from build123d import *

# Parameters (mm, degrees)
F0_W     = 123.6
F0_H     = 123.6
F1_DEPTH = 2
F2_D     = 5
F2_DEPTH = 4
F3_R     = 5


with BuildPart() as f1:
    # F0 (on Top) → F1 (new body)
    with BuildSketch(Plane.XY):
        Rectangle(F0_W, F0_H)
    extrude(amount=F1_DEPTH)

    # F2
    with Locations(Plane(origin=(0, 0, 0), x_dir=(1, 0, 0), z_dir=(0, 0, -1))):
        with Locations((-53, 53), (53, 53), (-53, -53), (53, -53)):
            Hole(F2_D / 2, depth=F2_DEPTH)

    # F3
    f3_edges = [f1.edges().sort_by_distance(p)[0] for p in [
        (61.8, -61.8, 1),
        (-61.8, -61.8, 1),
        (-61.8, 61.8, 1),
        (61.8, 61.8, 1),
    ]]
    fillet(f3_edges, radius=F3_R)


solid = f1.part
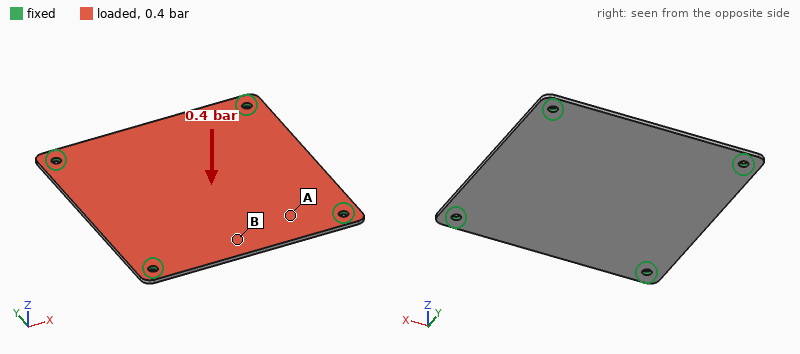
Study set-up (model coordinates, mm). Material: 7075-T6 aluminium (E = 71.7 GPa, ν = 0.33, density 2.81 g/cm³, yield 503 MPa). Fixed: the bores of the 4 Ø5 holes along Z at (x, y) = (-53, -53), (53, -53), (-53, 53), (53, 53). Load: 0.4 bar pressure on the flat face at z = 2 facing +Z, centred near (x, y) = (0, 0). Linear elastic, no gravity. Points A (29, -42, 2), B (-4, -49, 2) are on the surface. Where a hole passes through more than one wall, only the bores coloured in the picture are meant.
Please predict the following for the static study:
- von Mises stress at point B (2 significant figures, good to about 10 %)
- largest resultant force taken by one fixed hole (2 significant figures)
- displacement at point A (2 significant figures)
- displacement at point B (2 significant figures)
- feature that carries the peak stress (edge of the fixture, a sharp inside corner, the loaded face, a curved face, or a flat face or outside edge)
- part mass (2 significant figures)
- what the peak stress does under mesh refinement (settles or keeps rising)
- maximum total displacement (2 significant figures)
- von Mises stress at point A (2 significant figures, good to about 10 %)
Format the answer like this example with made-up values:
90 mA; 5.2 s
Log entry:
36 MPa; 150 N; 0.29 mm; 0.41 mm; edge of the fixture; 85 g; keeps rising; 0.71 mm; 15 MPa
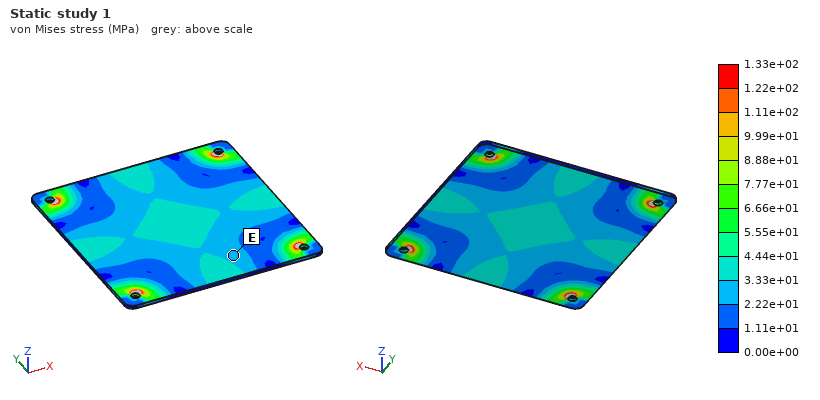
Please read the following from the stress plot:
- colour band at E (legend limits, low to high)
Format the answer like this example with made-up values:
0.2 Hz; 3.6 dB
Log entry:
2.22e+01 to 3.33e+01 MPa
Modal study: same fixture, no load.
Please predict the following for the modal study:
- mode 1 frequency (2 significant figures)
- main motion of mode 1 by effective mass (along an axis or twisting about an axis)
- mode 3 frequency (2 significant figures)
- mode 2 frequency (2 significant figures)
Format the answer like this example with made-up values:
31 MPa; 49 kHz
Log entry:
610 Hz; along Z; 1000 Hz; 1000 Hz
